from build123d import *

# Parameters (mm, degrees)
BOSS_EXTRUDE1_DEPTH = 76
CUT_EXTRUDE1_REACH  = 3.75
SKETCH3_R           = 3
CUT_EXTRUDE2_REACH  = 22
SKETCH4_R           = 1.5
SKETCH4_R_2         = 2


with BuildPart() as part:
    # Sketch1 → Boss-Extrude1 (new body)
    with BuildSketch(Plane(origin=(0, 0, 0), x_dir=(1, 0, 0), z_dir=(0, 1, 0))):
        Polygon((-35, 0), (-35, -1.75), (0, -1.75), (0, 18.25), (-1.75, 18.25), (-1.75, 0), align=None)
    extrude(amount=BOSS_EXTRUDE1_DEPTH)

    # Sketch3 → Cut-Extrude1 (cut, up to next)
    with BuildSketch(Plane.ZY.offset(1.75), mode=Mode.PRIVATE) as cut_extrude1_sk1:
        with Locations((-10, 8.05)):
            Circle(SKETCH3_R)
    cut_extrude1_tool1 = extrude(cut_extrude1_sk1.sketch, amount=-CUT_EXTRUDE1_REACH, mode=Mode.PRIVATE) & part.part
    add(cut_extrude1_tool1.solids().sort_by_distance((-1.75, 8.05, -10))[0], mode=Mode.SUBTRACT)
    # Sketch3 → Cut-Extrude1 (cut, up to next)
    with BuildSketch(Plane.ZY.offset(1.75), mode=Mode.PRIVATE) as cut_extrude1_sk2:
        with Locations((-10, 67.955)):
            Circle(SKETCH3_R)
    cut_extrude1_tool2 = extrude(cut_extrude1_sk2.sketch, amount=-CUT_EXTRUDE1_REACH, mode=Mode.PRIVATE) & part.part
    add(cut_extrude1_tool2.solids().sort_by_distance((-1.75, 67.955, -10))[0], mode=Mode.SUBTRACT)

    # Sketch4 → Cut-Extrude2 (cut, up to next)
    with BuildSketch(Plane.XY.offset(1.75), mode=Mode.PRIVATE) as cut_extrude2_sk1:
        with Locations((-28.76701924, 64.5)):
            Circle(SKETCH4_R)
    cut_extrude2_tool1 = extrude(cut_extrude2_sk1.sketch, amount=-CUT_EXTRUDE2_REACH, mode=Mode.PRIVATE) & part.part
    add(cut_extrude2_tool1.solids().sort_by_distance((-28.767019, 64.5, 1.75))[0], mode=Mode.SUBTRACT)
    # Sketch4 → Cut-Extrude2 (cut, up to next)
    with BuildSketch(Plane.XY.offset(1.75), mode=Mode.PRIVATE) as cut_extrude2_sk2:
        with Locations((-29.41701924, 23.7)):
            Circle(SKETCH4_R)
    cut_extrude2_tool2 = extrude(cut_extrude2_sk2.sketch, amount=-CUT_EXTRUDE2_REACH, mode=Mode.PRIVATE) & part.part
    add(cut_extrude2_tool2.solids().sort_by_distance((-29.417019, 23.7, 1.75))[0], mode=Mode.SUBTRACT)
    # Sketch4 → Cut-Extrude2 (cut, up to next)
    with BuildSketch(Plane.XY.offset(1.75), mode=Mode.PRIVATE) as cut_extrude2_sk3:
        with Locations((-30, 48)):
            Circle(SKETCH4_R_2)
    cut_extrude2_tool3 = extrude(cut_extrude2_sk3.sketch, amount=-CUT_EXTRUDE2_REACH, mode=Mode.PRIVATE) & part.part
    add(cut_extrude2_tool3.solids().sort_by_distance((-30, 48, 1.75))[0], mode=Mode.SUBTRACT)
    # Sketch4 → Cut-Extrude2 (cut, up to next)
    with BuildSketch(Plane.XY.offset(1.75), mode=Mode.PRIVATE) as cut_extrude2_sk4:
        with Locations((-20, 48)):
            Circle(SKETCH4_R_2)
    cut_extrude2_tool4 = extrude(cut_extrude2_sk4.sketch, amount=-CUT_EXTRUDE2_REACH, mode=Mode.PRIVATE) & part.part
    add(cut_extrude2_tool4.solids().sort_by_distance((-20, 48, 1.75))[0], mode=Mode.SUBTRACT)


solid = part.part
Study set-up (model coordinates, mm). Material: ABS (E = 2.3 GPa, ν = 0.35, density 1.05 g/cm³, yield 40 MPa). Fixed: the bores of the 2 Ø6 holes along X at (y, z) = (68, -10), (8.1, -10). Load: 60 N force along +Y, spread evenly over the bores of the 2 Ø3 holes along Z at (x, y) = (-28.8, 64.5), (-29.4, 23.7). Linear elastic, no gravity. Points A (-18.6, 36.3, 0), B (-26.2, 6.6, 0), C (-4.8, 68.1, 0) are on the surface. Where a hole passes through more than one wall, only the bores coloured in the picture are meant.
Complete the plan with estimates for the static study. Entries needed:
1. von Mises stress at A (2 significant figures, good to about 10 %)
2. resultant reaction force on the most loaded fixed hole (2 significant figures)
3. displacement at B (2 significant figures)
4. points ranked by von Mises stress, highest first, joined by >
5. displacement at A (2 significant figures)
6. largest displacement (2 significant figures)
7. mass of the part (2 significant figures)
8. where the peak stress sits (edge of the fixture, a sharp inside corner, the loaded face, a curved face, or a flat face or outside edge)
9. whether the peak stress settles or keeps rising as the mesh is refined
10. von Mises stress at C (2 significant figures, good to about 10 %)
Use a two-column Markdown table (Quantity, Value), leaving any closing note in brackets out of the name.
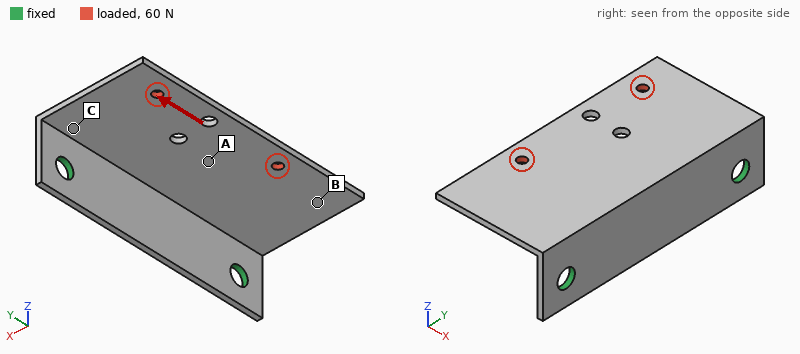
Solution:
| Quantity | Value |
|---|---|
| von Mises stress at A | 2.7 MPa |
| resultant reaction force on the most loaded fixed hole | 42 N |
| displacement at B | 0.66 mm |
| points ranked by von Mises stress, highest first, joined by > | C > A > B |
| displacement at A | 0.18 mm |
| largest displacement | 0.92 mm |
| mass of the part | 7.3 g |
| where the peak stress sits | edge of the fixture |
| whether the peak stress settles or keeps rising as the mesh is refined | keeps rising |
| von Mises stress at C | 5.3 MPa |
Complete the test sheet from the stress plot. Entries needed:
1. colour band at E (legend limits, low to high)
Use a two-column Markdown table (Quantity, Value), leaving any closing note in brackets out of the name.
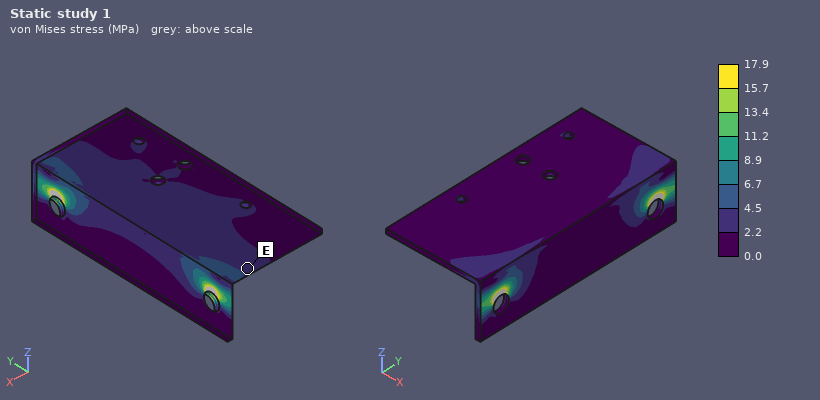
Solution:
| Quantity | Value |
|---|---|
| colour band at E | 2.2 to 4.5 MPa |
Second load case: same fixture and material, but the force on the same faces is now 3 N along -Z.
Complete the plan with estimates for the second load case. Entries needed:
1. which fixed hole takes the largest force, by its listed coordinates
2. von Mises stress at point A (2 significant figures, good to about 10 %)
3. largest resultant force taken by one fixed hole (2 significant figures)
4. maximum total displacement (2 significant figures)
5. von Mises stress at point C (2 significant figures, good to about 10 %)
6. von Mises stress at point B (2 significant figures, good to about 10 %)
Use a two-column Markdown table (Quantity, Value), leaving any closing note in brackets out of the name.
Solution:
| Quantity | Value |
|---|---|
| which fixed hole takes the largest force, by its listed coordinates | (68, -10) |
| von Mises stress at point A | 0.73 MPa |
| largest resultant force taken by one fixed hole | 1.8 N |
| maximum total displacement | 0.85 mm |
| von Mises stress at point C | 1.9 MPa |
| von Mises stress at point B | 0.42 MPa |
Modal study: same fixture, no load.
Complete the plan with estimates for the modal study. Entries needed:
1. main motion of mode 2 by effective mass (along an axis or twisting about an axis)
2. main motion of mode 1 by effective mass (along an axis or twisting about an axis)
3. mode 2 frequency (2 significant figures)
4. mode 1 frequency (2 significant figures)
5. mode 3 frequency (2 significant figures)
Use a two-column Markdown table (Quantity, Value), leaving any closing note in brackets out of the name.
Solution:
| Quantity | Value |
|---|---|
| main motion of mode 2 by effective mass | twisting about X |
| main motion of mode 1 by effective mass | along Z |
| mode 2 frequency | 420 Hz |
| mode 1 frequency | 240 Hz |
| mode 3 frequency | 850 Hz |
